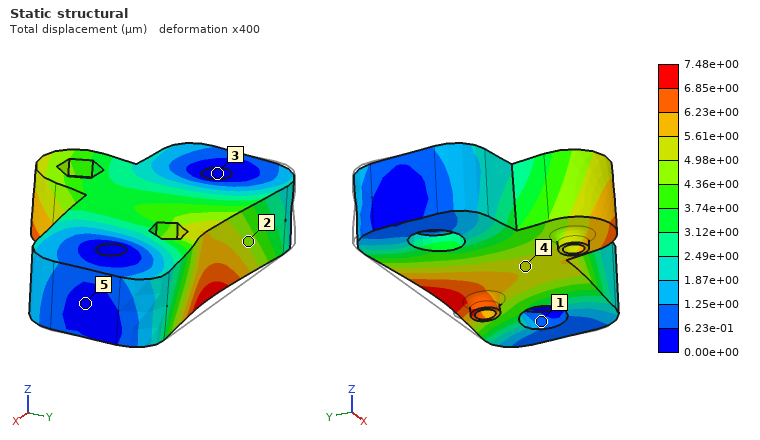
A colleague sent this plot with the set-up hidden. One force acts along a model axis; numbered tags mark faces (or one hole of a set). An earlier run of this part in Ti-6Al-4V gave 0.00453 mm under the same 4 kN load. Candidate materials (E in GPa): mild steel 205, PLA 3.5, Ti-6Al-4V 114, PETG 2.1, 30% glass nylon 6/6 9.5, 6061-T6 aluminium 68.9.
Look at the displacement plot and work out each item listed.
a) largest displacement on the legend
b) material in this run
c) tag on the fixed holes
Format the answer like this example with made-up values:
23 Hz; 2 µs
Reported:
7.48e+00 µm; 6061-T6 aluminium; 3
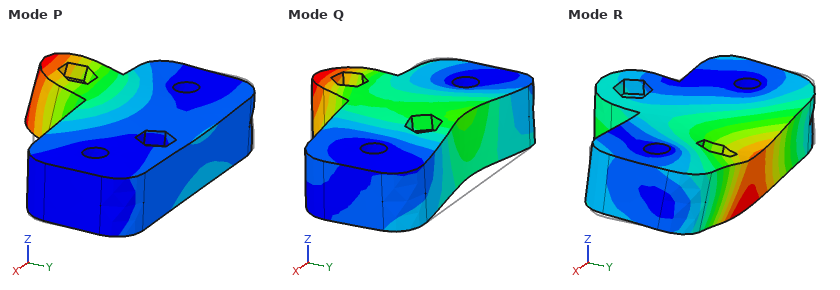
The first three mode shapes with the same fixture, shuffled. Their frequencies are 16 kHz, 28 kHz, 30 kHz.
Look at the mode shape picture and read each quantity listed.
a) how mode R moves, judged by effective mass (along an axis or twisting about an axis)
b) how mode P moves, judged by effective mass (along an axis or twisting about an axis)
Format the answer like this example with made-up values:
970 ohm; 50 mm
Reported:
along Z; along Z
